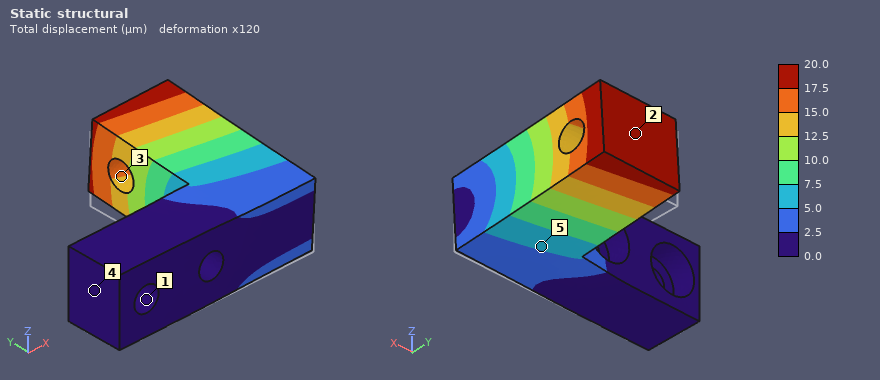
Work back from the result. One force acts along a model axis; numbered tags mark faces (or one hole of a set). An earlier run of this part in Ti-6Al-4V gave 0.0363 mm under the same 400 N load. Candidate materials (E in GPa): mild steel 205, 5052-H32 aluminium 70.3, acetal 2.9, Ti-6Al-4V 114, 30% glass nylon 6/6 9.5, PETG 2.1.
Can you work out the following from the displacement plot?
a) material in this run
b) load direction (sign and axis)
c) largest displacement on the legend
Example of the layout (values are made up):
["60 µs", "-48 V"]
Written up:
["mild steel", "+Z", "20.0 µm"]
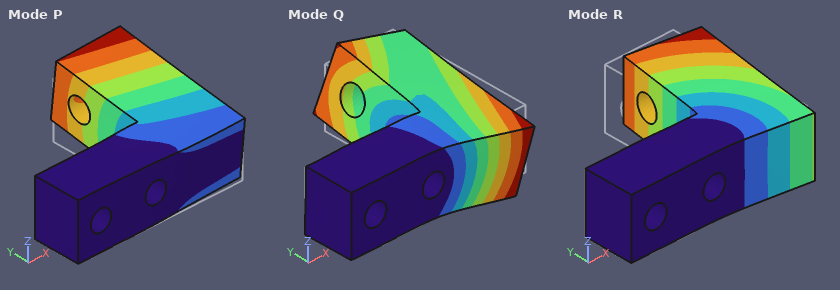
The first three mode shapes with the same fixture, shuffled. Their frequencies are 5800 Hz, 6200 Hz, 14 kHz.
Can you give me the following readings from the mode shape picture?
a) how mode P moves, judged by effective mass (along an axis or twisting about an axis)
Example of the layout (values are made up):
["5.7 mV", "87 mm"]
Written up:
["along Z"]
